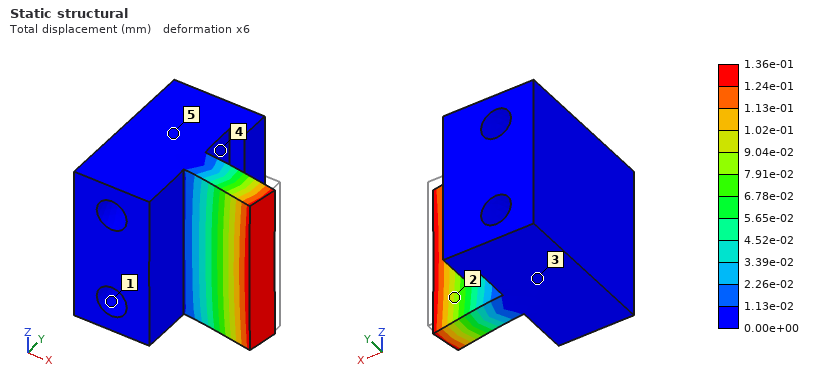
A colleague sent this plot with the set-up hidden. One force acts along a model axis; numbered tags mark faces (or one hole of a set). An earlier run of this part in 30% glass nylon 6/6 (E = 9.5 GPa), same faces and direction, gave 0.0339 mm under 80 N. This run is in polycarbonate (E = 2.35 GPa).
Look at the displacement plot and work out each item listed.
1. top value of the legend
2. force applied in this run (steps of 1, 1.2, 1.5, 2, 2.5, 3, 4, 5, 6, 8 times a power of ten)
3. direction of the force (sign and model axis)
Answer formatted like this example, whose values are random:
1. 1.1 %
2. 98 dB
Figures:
1. 1.36e-01 mm
2. 80 N
3. -Y
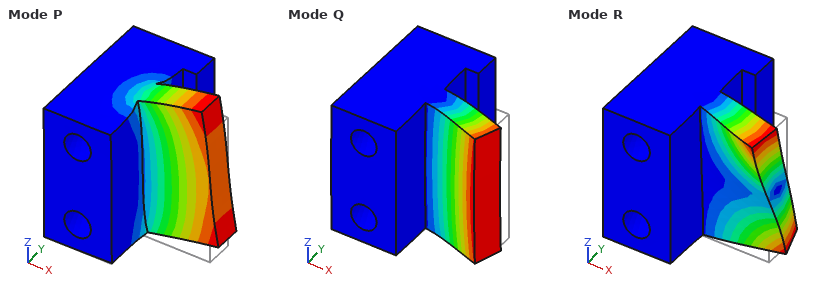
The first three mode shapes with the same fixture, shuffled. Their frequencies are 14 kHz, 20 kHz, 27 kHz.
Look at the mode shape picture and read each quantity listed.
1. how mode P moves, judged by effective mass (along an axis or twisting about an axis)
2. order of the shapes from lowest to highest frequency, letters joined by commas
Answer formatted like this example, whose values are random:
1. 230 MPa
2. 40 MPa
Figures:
1. along Z
2. Q, R, P
